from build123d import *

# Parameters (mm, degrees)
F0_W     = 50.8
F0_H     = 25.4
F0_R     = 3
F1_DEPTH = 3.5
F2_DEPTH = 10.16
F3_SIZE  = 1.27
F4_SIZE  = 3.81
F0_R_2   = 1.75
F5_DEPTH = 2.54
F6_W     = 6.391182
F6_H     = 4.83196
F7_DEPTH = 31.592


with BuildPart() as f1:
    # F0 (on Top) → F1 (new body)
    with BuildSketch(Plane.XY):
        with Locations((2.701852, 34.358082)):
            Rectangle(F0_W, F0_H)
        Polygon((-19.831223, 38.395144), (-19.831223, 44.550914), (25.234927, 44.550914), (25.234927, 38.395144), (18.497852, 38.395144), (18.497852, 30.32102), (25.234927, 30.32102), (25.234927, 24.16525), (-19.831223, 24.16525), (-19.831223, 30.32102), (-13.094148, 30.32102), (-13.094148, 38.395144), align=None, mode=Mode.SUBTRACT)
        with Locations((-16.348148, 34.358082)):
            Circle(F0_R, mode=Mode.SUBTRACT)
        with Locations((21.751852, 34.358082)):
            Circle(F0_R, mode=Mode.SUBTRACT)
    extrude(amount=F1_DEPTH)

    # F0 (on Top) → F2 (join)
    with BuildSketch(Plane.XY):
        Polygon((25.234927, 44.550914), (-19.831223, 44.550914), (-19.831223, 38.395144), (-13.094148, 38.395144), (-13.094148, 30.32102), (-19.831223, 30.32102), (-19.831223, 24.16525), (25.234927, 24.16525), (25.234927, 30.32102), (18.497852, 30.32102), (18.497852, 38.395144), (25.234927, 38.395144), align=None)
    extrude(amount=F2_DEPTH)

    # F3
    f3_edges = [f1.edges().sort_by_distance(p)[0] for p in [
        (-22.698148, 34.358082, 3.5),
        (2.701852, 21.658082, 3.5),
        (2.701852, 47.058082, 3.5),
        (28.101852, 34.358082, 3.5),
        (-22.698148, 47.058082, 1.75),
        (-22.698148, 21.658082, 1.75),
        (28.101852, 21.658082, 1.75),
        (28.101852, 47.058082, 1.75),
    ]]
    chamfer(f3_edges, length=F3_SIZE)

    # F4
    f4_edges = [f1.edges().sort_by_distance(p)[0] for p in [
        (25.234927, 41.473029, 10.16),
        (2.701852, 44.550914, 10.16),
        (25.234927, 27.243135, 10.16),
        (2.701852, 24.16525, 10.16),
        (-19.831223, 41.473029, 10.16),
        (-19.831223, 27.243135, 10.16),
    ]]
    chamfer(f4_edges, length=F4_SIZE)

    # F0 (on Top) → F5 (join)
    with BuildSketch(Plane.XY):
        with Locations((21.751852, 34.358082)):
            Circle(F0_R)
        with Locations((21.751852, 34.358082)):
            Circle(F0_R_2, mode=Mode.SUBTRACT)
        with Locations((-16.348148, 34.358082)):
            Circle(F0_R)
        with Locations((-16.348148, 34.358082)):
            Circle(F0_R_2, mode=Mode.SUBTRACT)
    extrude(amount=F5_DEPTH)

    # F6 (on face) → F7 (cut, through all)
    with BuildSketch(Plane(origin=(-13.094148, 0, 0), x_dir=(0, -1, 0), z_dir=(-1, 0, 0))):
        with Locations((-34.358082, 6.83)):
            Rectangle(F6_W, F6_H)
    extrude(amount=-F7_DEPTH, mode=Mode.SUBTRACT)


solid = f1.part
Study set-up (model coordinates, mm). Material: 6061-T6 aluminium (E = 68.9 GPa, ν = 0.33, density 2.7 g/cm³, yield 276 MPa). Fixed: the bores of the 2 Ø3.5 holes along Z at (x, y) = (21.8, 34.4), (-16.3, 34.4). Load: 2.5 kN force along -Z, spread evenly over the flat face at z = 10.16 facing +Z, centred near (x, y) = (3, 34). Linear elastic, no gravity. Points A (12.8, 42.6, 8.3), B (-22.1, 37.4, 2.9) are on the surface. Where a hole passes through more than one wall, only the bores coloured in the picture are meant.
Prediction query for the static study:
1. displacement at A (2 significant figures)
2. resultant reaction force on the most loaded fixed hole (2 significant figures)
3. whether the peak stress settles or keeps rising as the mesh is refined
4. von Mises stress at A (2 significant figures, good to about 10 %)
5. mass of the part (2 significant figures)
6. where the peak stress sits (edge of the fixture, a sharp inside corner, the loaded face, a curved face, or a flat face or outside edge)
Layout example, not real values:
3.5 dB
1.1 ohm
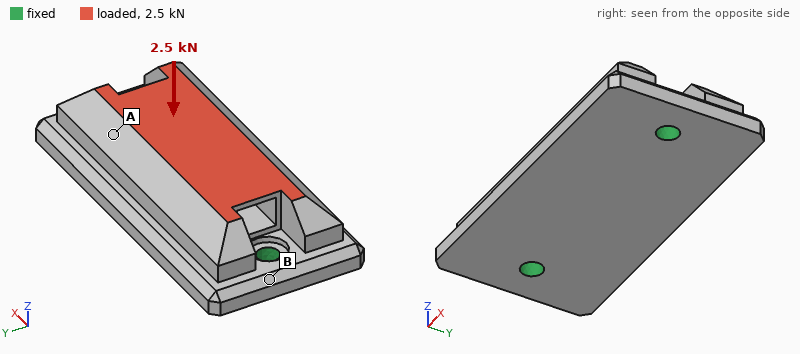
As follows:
18 µm
1.6 kN
keeps rising
24 MPa
21 g
edge of the fixture
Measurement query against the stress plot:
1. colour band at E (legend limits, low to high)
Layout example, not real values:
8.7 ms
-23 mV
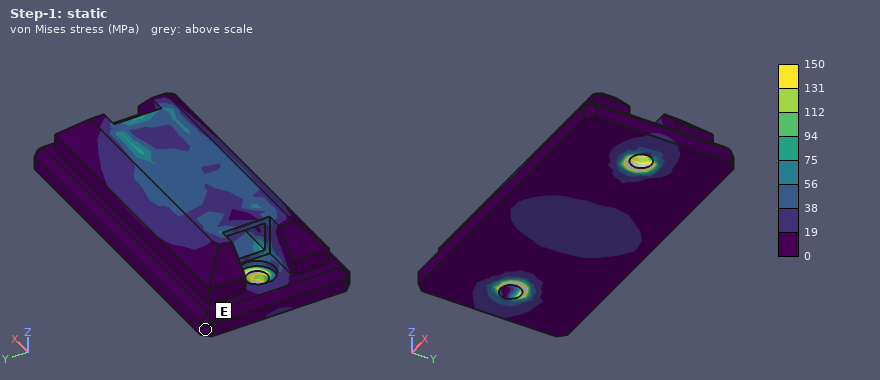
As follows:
0 to 19 MPa
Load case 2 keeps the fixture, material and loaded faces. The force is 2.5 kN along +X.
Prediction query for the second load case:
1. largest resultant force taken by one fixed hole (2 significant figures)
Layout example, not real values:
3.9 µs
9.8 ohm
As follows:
1.4 kN
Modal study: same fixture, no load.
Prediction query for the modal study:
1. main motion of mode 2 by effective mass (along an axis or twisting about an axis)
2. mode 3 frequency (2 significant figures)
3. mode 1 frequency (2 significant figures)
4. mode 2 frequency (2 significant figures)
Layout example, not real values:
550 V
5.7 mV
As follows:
along Z
21 kHz
6700 Hz
14 kHz
